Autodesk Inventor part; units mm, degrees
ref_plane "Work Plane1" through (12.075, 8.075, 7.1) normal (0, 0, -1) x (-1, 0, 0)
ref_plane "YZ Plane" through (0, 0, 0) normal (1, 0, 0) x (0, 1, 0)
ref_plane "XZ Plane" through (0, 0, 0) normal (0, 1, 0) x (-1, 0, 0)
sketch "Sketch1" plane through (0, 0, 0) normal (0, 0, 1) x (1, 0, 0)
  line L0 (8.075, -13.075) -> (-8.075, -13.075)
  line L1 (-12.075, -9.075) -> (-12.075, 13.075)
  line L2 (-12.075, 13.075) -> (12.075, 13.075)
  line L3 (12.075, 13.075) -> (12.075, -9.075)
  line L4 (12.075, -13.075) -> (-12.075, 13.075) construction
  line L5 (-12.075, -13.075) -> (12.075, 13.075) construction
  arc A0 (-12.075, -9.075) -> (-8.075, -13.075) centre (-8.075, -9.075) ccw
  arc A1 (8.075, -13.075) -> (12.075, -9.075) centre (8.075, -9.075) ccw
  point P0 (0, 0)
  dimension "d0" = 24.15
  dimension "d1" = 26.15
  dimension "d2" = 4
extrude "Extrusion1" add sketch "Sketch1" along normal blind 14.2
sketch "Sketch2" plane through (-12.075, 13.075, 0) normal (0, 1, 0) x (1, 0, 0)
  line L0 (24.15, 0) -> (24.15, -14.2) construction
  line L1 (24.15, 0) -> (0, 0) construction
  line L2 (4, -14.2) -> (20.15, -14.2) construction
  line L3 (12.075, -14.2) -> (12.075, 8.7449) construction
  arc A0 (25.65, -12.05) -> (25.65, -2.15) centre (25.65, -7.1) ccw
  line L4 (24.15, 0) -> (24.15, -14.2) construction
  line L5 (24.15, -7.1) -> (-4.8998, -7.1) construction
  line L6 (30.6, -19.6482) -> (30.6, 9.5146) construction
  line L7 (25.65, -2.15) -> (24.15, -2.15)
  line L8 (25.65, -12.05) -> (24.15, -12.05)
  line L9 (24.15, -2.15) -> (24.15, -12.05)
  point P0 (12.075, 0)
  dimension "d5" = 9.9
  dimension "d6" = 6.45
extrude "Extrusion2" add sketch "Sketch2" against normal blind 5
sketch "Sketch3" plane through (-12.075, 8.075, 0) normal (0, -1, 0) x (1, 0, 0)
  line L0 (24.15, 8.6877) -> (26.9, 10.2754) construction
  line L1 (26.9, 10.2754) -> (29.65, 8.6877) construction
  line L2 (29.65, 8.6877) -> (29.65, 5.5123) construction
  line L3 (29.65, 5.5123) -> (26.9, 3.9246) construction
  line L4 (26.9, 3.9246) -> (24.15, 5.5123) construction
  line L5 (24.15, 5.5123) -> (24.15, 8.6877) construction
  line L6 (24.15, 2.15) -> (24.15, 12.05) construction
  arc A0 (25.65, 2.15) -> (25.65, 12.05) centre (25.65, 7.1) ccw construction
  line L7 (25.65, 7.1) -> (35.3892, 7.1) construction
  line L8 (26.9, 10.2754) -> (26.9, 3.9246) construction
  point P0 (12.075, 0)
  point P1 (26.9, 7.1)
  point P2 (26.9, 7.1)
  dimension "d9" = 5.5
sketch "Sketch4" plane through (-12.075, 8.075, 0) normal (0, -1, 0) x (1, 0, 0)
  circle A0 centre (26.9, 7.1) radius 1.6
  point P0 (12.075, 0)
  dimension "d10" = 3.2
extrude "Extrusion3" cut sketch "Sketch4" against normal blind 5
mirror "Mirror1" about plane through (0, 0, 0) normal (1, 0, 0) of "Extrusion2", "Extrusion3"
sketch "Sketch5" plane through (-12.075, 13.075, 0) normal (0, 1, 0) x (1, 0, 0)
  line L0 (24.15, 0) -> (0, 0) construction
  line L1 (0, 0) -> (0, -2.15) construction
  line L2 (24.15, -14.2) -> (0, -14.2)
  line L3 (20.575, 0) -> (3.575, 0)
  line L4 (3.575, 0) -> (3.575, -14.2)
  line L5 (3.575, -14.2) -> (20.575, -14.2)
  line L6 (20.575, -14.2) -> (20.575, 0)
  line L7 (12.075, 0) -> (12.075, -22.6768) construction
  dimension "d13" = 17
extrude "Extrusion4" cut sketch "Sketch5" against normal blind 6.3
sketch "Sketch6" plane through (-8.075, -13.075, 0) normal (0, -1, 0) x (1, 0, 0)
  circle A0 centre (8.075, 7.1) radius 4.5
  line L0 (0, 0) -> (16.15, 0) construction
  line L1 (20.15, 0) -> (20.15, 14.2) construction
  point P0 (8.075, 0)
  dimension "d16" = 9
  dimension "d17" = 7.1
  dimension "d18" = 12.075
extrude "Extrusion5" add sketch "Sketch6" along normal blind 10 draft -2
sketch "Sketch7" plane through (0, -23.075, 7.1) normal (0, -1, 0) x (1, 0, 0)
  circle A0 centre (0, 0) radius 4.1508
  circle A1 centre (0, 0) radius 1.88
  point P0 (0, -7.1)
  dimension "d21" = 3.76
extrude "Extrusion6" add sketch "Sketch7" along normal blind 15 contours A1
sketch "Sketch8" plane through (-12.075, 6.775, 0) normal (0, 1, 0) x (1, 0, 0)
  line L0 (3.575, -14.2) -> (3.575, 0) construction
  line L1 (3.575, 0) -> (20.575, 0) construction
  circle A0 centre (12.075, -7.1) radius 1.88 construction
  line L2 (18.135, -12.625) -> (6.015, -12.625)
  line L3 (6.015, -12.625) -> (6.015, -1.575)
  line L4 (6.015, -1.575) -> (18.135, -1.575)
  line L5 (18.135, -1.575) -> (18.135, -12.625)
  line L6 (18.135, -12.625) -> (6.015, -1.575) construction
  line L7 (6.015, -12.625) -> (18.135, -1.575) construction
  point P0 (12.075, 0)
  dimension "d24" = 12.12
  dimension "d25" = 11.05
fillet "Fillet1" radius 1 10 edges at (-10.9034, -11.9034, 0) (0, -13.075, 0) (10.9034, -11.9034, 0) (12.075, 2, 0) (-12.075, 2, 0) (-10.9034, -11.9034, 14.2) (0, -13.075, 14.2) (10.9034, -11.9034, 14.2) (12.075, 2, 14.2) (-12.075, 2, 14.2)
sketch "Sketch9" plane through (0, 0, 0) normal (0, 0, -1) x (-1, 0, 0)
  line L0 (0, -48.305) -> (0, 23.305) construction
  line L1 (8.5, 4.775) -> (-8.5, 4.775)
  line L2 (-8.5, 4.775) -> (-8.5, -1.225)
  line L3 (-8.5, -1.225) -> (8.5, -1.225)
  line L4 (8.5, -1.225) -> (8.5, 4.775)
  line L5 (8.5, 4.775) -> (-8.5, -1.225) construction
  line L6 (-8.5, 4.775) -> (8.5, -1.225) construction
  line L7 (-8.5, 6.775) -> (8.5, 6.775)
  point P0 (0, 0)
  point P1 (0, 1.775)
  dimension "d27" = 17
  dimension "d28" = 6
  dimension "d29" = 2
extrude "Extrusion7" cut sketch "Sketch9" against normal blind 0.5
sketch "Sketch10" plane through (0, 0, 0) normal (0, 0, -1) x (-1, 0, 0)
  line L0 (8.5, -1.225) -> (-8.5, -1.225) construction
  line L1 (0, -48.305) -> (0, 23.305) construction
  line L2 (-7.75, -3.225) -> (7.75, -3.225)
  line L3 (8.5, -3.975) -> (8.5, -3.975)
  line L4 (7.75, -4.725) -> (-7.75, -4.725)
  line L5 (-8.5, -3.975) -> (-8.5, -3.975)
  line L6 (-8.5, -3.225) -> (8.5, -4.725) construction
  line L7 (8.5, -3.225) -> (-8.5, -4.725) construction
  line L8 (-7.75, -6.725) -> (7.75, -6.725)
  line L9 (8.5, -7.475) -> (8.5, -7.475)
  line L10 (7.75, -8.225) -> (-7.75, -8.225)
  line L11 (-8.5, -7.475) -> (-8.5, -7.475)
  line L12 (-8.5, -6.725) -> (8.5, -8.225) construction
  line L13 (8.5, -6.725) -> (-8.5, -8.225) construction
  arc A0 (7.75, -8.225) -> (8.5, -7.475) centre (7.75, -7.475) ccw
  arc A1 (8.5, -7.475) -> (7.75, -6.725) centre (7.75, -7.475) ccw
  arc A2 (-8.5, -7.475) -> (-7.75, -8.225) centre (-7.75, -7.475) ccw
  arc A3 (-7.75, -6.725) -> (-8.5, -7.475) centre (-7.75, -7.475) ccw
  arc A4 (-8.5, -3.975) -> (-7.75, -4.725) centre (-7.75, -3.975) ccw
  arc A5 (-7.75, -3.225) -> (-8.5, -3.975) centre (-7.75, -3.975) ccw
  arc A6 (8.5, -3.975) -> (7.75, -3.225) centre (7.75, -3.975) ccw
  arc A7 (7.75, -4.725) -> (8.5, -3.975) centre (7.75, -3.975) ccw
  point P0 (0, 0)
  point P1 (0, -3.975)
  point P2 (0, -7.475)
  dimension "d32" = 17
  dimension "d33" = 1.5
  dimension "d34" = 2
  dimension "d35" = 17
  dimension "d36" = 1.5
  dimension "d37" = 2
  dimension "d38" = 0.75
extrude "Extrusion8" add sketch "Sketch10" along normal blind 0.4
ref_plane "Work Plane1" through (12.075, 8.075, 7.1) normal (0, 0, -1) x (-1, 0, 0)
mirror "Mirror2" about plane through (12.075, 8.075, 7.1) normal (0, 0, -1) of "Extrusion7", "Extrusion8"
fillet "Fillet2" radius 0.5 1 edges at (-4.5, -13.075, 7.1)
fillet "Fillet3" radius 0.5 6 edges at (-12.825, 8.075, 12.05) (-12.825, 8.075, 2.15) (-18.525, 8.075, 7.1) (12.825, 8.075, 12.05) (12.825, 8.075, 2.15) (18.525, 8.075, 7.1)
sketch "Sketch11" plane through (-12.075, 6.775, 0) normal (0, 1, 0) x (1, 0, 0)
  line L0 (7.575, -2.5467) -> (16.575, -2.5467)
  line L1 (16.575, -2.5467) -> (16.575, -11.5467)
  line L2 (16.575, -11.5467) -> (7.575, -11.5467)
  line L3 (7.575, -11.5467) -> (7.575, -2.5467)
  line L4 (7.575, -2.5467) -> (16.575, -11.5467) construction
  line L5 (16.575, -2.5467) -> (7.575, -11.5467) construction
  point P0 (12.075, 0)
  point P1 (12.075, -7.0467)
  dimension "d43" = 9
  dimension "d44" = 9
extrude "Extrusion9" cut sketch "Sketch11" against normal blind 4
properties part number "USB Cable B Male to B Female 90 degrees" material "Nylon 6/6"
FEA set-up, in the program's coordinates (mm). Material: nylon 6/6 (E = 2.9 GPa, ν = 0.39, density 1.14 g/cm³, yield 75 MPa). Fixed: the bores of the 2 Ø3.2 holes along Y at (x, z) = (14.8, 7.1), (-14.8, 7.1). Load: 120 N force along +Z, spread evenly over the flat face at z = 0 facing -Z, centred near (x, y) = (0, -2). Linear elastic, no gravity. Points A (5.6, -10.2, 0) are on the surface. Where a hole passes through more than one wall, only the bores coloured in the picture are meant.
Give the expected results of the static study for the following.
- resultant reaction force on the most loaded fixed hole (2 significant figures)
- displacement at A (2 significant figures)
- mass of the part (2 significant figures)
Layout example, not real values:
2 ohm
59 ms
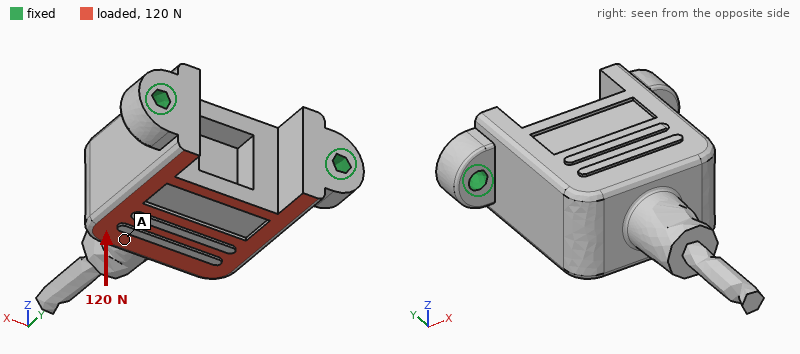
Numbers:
60 N
0.23 mm
9.3 g
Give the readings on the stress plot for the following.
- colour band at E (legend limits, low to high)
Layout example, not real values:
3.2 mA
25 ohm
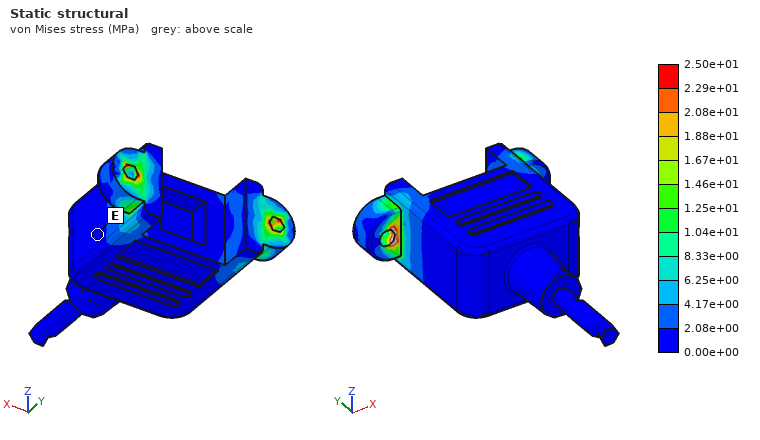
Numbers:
0.00e+00 to 2.08e+00 MPa
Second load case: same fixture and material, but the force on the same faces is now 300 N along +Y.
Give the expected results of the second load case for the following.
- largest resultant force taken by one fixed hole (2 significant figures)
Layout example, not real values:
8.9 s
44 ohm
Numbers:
160 N
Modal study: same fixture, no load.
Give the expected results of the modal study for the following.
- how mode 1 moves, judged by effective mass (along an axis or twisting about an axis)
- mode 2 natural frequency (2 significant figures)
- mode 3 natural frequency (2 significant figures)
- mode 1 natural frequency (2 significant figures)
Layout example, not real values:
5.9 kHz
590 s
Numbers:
along Z
3000 Hz
3300 Hz
1200 Hz
